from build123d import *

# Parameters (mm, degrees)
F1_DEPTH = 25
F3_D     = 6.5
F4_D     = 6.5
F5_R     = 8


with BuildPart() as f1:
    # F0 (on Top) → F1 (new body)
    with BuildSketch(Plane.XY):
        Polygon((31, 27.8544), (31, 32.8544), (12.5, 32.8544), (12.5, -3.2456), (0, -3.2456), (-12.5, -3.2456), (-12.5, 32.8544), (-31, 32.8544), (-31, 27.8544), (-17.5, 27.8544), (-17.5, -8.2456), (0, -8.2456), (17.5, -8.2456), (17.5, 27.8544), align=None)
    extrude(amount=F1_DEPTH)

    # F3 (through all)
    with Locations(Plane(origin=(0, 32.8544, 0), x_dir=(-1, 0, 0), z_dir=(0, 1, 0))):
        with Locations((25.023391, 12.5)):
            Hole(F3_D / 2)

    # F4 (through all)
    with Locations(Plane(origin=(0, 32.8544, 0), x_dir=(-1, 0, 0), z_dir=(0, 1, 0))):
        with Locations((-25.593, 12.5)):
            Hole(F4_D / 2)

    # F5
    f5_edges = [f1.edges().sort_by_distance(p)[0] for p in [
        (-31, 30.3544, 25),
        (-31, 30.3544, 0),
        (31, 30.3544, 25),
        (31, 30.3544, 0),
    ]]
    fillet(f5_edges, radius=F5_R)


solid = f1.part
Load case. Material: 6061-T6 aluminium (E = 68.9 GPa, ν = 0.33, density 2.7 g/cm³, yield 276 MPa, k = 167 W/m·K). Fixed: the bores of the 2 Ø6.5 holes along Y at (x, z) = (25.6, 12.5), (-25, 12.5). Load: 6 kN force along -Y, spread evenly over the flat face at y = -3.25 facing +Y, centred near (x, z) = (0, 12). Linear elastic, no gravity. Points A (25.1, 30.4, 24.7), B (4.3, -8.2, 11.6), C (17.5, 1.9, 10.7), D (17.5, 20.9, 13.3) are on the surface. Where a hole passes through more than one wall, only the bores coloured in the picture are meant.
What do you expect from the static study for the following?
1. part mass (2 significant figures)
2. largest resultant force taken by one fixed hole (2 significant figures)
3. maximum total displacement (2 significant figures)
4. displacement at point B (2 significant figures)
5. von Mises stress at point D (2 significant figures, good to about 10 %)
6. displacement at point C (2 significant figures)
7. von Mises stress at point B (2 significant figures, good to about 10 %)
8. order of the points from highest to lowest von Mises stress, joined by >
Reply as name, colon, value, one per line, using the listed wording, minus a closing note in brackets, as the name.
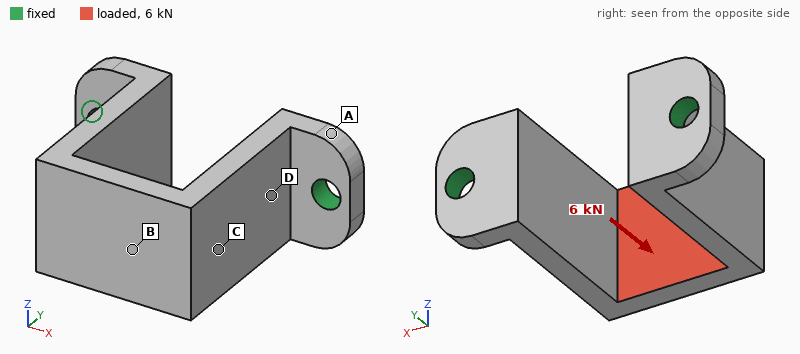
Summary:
part mass: 44 g
largest resultant force taken by one fixed hole: 3.1 kN
maximum total displacement: 0.11 mm
displacement at point B: 0.090 mm
von Mises stress at point D: 72 MPa
displacement at point C: 0.043 mm
von Mises stress at point B: 100 MPa
order of the points from highest to lowest von Mises stress, joined by >: B > D > C > A
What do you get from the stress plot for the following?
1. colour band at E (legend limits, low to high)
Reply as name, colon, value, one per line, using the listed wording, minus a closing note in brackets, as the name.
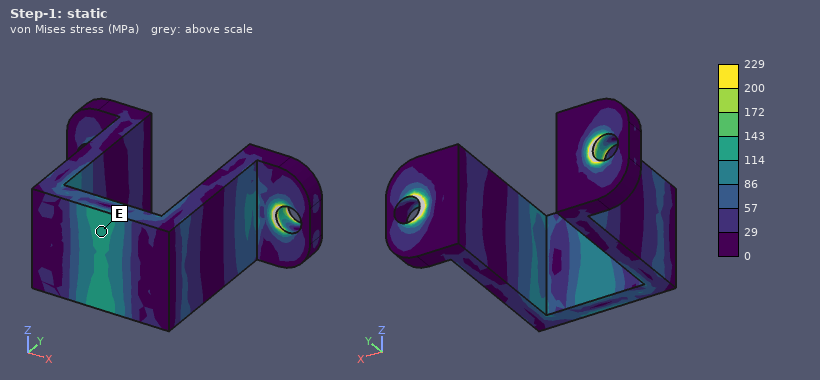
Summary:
colour band at E: 114 to 143 MPa
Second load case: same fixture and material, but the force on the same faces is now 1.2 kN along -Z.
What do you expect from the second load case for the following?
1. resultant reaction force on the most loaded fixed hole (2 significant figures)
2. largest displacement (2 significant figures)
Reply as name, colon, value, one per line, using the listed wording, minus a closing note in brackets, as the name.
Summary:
resultant reaction force on the most loaded fixed hole: 610 N
largest displacement: 0.25 mm
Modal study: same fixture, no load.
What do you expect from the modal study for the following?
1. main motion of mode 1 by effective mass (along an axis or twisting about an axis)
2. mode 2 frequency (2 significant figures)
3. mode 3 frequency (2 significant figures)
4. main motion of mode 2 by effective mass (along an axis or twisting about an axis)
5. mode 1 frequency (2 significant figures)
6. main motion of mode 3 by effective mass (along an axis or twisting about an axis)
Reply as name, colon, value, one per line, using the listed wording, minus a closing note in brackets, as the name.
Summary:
main motion of mode 1 by effective mass: along Z
mode 2 frequency: 2800 Hz
mode 3 frequency: 4600 Hz
main motion of mode 2 by effective mass: along X
mode 1 frequency: 2600 Hz
main motion of mode 3 by effective mass: twisting about Y
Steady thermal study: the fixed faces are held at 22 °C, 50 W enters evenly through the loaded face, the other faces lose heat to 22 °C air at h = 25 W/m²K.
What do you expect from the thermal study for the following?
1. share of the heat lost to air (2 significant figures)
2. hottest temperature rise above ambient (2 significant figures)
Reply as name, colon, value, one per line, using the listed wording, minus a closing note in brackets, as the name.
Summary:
share of the heat lost to air: 9.8 %
hottest temperature rise above ambient: 57 K
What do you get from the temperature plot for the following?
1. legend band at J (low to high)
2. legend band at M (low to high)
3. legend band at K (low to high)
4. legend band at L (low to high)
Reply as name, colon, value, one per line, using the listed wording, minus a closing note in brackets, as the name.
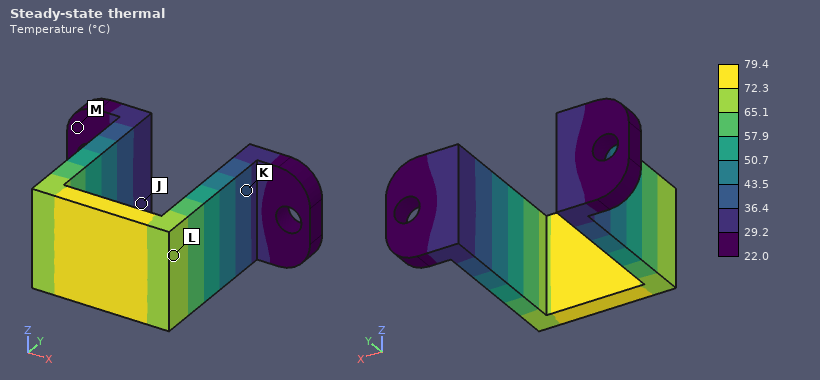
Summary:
legend band at J: 29.2 to 36.4 °C
legend band at M: 22.0 to 29.2 °C
legend band at K: 36.4 to 43.5 °C
legend band at L: 65.1 to 72.3 °C
